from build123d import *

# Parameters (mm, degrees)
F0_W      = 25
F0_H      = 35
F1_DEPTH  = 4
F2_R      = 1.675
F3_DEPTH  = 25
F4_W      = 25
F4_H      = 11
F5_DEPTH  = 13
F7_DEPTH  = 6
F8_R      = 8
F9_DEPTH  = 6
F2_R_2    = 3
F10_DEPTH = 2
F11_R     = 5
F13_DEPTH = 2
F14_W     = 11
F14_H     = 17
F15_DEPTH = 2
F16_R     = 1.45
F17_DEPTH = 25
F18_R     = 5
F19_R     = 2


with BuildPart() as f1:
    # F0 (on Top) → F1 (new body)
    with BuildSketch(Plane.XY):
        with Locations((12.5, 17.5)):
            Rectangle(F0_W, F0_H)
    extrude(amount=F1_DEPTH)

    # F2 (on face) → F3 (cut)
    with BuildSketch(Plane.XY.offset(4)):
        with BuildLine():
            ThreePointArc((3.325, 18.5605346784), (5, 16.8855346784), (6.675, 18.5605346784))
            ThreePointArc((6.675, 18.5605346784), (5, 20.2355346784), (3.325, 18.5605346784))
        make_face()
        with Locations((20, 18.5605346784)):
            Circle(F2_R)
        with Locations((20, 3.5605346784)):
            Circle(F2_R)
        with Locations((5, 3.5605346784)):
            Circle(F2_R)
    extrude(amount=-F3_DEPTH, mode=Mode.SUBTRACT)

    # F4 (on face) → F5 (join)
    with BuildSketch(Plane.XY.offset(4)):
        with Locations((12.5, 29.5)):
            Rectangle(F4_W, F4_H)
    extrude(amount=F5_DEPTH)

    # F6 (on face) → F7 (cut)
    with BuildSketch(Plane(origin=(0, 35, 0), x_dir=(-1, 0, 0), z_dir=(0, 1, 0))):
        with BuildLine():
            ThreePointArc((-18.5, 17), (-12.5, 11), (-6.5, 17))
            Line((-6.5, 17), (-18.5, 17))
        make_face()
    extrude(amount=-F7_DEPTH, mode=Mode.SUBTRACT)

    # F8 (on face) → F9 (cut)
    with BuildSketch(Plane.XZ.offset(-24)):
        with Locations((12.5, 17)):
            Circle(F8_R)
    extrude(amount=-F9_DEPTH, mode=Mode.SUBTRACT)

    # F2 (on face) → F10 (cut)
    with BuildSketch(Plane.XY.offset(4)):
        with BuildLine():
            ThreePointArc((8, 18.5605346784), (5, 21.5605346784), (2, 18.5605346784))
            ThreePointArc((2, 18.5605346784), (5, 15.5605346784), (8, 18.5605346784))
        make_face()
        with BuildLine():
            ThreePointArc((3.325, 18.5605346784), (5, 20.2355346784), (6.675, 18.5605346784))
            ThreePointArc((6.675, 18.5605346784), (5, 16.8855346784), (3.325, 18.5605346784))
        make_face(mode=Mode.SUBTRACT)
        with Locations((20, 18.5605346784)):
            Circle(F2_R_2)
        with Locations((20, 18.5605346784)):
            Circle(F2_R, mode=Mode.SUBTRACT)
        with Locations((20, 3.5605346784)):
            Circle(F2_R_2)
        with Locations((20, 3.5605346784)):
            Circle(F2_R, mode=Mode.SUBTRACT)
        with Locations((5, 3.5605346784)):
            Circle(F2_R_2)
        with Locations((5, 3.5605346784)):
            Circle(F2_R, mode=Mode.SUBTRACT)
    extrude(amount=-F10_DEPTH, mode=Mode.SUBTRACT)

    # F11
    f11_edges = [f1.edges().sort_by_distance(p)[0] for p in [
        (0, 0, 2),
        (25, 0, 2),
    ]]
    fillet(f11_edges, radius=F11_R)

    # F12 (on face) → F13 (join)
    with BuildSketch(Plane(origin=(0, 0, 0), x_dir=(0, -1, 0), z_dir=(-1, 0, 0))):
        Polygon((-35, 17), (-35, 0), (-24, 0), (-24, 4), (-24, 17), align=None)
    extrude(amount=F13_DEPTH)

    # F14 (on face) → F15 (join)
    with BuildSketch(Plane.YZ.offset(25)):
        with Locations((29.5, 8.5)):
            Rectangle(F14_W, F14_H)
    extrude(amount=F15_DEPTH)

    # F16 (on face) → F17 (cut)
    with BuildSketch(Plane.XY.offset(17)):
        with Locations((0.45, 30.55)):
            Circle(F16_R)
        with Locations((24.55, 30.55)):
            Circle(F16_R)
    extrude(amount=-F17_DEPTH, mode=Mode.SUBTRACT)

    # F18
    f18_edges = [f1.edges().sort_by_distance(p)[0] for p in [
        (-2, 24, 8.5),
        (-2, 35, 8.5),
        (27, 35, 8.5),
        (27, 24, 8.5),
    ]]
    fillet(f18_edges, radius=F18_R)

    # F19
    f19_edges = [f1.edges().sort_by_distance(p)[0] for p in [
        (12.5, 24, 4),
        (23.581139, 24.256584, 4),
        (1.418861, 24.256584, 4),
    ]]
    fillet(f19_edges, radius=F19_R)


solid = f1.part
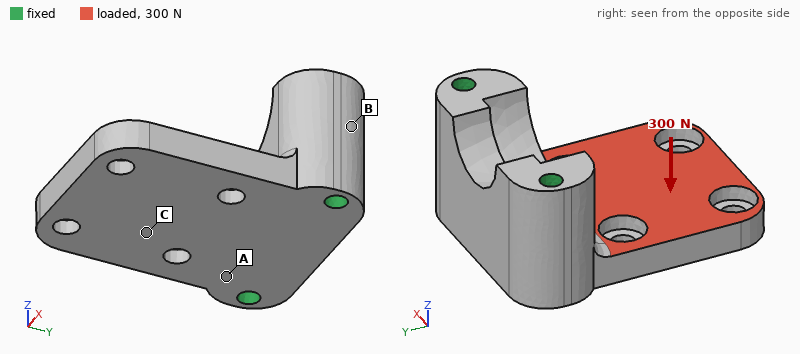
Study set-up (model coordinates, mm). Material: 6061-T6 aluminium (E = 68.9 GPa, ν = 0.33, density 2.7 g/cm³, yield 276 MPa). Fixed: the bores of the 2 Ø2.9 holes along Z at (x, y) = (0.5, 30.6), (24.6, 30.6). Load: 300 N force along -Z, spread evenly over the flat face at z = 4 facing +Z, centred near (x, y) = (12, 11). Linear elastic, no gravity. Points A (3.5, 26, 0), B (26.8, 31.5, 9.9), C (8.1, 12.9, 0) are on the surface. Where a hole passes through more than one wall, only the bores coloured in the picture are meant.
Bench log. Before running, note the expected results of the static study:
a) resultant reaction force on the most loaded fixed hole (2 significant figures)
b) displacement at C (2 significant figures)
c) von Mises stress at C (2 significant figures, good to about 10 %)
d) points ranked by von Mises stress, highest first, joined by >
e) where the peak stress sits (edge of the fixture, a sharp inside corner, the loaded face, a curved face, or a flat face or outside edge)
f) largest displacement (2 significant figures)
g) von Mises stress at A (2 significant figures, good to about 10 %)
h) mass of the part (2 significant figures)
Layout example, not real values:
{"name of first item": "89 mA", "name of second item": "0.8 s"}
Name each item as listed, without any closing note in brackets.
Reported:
{"resultant reaction force on the most loaded fixed hole": "150 N", "displacement at C": "36 µm", "von Mises stress at C": "15 MPa", "points ranked by von Mises stress, highest first, joined by >": "A > C > B", "where the peak stress sits": "the loaded face", "largest displacement": "95 µm", "von Mises stress at A": "27 MPa", "mass of the part": "16 g"}
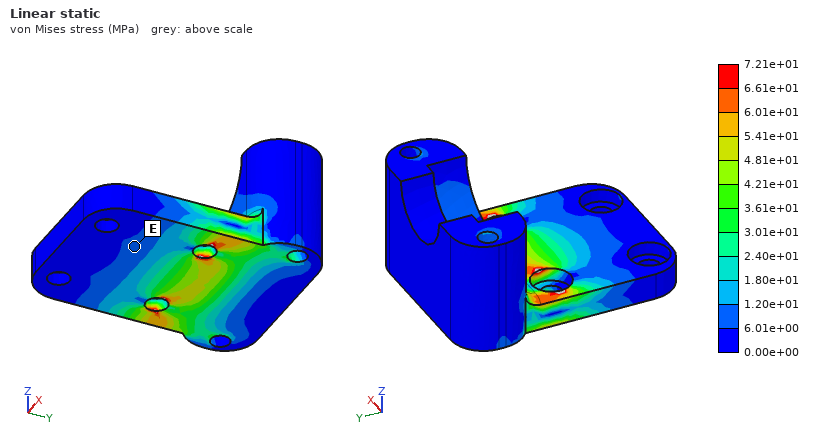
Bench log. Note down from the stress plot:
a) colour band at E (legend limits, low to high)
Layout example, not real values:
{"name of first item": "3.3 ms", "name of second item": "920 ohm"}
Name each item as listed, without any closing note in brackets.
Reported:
{"colour band at E": "6.01e+00 to 1.20e+01 MPa"}
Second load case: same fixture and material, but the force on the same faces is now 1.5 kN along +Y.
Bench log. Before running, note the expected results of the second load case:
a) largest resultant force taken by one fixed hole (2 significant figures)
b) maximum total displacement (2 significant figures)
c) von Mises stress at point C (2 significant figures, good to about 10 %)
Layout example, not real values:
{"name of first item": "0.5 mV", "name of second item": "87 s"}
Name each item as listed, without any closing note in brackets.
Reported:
{"largest resultant force taken by one fixed hole": "780 N", "maximum total displacement": "96 µm", "von Mises stress at point C": "17 MPa"}
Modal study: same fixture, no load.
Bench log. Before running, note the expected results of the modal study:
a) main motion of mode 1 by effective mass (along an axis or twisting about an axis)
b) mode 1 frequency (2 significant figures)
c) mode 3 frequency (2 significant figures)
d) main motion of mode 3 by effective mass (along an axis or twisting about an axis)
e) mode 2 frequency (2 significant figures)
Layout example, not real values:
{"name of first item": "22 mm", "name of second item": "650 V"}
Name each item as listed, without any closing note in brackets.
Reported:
{"main motion of mode 1 by effective mass": "along Z", "mode 1 frequency": "5000 Hz", "mode 3 frequency": "18 kHz", "main motion of mode 3 by effective mass": "along X", "mode 2 frequency": "12 kHz"}
